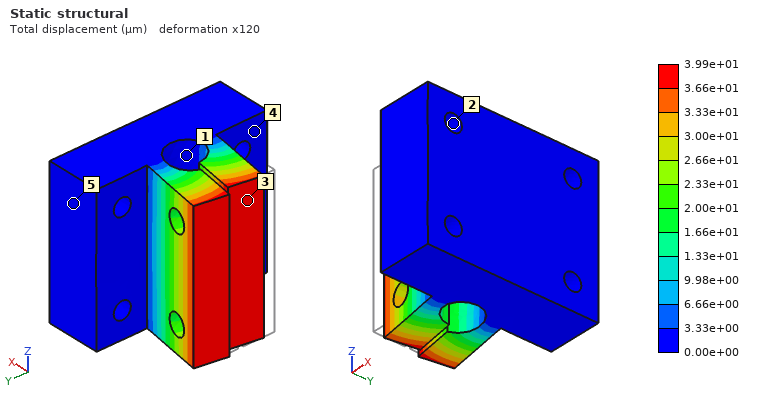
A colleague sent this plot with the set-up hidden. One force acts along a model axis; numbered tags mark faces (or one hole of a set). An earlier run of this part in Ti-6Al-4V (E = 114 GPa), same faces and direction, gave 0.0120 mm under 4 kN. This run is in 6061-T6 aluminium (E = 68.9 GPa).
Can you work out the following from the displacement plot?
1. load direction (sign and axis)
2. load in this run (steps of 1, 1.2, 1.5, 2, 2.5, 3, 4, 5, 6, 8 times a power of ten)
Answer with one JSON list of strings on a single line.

["+Y", "8 kN"]
